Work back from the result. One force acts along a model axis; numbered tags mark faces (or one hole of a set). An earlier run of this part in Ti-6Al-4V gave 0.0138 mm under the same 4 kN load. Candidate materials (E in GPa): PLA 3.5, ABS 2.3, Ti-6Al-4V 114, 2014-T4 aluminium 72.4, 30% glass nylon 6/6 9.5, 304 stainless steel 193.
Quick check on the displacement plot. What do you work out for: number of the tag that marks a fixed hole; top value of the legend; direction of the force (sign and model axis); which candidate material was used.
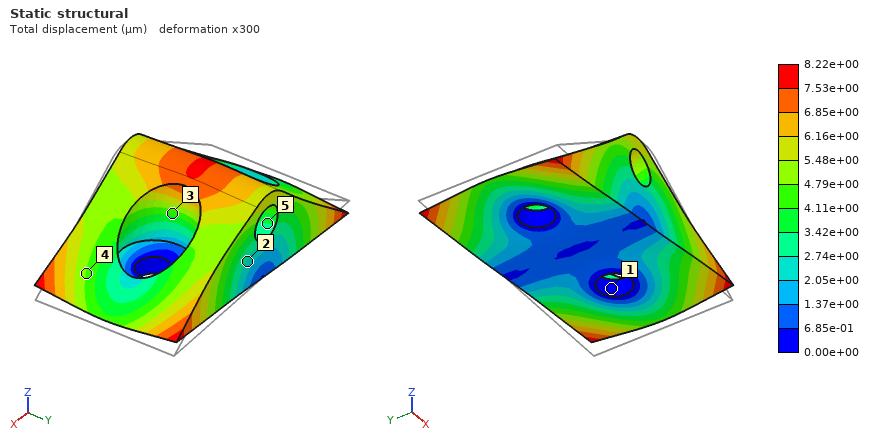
1
8.22e+00 µm
-X
304 stainless steel
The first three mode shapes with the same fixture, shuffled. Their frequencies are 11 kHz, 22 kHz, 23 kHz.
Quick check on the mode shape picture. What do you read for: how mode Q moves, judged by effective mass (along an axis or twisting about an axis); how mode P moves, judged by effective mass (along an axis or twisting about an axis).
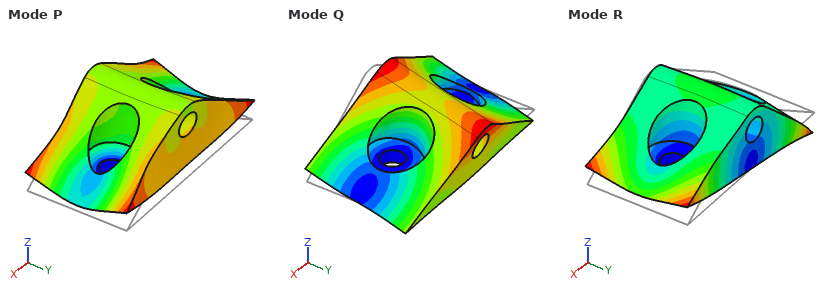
along Y
along Z
